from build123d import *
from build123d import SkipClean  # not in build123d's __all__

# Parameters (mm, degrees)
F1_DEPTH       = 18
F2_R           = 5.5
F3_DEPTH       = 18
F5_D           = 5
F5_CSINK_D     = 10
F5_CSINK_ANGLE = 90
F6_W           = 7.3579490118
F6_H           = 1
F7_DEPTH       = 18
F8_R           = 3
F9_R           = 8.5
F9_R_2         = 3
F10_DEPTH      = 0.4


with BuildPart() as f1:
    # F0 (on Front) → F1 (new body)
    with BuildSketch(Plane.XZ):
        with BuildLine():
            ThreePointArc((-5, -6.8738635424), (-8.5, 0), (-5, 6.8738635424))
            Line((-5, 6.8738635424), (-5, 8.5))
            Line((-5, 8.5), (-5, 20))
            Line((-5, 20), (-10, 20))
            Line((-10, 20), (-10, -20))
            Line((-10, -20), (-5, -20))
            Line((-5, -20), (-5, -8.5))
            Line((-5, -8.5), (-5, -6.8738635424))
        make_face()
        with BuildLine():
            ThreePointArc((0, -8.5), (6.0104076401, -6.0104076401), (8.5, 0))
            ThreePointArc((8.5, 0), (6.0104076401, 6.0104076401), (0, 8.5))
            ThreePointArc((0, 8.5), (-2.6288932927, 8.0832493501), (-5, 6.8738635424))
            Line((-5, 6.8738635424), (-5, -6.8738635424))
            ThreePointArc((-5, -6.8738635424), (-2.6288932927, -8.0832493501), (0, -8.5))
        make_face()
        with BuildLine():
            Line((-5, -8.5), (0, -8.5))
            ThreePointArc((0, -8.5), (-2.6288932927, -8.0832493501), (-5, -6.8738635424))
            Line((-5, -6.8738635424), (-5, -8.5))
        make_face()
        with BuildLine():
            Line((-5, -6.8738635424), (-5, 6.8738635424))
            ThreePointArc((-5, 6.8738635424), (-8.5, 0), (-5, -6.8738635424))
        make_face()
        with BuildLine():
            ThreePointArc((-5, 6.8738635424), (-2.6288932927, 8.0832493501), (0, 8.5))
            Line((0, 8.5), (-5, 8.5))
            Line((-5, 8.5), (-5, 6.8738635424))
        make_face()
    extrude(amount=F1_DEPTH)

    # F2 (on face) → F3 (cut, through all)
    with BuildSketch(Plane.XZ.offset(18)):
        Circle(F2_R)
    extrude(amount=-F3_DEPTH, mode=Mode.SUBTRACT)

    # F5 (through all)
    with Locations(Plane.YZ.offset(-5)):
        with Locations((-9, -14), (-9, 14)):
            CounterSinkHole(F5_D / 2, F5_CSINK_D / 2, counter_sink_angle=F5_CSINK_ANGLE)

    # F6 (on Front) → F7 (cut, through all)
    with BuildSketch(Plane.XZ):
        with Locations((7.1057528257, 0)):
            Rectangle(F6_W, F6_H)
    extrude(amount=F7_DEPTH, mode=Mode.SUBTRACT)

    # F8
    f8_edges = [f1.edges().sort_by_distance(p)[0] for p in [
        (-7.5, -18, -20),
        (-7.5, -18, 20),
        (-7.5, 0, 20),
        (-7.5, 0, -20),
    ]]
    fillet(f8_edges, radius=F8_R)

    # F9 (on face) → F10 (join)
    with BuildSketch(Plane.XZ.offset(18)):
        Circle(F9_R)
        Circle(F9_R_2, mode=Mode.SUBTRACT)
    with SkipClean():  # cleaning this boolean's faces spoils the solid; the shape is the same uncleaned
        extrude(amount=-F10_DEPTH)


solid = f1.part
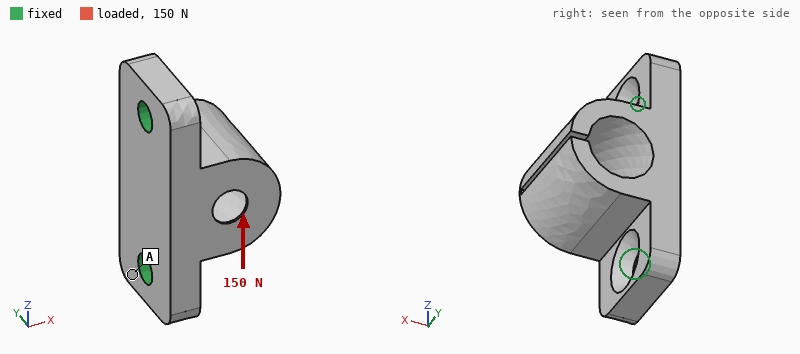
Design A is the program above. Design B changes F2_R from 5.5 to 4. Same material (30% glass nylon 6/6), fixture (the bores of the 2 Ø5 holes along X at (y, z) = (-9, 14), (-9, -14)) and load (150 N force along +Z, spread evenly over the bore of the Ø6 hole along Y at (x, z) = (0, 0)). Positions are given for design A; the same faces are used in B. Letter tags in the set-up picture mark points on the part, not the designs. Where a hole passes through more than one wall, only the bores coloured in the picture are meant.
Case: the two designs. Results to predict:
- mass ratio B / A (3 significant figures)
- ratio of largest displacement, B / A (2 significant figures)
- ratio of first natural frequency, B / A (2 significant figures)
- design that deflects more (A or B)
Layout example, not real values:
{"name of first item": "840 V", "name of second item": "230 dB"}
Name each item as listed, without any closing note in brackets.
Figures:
{"mass ratio B / A": "1.15", "ratio of largest displacement, B / A": "0.63", "ratio of first natural frequency, B / A": "0.90", "design that deflects more": "A"}
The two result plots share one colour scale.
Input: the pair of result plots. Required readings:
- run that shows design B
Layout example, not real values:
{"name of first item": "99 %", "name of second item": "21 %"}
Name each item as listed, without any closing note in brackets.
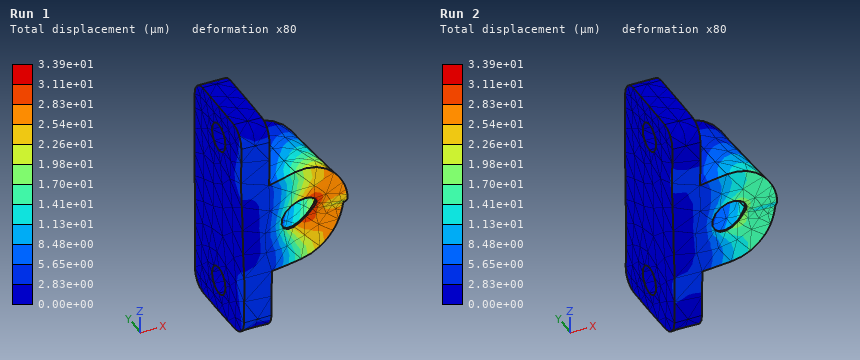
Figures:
{"run that shows design B": "Run 2"}
